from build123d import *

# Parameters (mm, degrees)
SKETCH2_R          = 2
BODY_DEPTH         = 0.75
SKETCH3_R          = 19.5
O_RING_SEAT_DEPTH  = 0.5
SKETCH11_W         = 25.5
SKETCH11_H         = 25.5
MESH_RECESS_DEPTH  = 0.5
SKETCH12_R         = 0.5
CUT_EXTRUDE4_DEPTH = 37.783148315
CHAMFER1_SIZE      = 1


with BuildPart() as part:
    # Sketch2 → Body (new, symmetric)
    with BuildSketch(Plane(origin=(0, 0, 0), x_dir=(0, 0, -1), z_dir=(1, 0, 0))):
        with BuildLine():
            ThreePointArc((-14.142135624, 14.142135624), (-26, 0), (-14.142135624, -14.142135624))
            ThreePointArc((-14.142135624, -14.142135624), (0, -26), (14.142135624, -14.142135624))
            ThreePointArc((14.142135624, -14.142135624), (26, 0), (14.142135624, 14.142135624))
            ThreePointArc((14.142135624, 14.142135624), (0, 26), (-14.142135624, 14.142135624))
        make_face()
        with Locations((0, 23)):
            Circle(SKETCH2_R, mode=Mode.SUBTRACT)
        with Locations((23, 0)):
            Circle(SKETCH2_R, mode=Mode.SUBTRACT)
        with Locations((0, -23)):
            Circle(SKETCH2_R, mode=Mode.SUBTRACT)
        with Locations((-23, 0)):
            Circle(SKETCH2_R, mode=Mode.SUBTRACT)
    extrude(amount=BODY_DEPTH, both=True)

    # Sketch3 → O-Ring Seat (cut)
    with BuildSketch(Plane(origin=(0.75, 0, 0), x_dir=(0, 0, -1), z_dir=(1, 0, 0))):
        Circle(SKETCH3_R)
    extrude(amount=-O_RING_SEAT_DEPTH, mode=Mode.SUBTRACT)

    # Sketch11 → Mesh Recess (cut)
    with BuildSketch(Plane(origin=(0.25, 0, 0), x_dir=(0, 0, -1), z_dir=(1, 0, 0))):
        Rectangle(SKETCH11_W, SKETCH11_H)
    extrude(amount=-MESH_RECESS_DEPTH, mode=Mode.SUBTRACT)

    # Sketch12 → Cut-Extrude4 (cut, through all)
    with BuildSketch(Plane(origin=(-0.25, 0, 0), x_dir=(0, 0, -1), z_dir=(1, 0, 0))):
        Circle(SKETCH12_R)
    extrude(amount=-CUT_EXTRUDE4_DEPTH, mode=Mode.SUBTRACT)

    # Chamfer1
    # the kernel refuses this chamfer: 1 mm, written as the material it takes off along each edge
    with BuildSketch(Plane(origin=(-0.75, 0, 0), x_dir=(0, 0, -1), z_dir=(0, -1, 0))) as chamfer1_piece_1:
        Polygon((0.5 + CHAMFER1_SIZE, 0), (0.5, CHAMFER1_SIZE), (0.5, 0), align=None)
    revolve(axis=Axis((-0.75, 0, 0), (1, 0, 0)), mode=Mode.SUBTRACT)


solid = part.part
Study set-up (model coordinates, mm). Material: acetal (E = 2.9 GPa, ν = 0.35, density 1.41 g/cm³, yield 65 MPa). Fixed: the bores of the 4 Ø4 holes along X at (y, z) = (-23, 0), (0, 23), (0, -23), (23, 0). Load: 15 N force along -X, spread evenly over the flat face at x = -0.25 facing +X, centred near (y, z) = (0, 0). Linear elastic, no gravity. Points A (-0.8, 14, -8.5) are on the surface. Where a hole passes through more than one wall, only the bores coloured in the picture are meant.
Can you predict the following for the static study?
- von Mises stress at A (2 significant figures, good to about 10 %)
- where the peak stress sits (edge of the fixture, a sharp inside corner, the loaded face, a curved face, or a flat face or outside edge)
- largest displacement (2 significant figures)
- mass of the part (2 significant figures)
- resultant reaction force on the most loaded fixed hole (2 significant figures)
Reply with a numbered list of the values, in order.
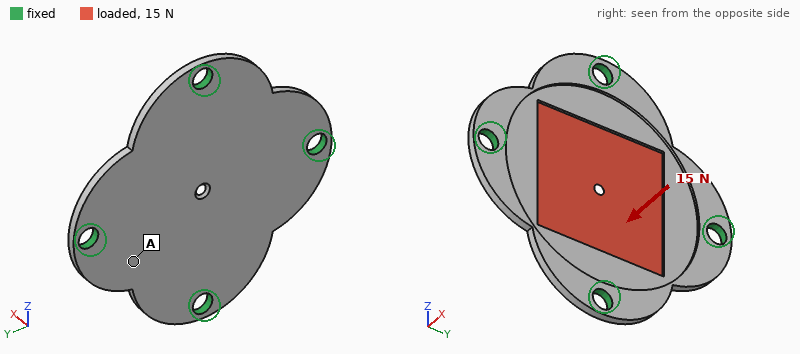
1. 3.8 MPa
2. the loaded face
3. 0.73 mm
4. 2.4 g
5. 14 N
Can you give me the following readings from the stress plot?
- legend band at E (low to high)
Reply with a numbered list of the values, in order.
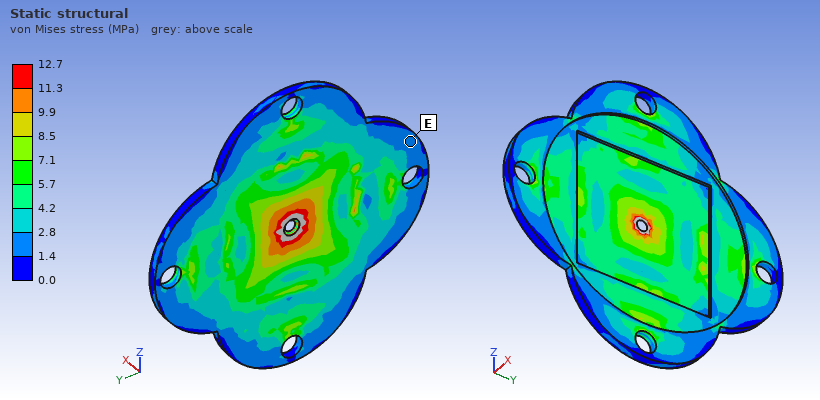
1. 1.4 to 2.8 MPa
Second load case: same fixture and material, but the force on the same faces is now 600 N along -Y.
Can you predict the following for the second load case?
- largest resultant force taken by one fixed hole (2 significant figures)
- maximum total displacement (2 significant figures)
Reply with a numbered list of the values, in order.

1. 190 N
2. 0.41 mm
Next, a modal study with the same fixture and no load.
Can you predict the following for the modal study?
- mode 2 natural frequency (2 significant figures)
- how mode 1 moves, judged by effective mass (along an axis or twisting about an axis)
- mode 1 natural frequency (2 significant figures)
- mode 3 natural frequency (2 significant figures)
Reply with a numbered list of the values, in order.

1. 2200 Hz
2. along X
3. 1400 Hz
4. 2200 Hz
